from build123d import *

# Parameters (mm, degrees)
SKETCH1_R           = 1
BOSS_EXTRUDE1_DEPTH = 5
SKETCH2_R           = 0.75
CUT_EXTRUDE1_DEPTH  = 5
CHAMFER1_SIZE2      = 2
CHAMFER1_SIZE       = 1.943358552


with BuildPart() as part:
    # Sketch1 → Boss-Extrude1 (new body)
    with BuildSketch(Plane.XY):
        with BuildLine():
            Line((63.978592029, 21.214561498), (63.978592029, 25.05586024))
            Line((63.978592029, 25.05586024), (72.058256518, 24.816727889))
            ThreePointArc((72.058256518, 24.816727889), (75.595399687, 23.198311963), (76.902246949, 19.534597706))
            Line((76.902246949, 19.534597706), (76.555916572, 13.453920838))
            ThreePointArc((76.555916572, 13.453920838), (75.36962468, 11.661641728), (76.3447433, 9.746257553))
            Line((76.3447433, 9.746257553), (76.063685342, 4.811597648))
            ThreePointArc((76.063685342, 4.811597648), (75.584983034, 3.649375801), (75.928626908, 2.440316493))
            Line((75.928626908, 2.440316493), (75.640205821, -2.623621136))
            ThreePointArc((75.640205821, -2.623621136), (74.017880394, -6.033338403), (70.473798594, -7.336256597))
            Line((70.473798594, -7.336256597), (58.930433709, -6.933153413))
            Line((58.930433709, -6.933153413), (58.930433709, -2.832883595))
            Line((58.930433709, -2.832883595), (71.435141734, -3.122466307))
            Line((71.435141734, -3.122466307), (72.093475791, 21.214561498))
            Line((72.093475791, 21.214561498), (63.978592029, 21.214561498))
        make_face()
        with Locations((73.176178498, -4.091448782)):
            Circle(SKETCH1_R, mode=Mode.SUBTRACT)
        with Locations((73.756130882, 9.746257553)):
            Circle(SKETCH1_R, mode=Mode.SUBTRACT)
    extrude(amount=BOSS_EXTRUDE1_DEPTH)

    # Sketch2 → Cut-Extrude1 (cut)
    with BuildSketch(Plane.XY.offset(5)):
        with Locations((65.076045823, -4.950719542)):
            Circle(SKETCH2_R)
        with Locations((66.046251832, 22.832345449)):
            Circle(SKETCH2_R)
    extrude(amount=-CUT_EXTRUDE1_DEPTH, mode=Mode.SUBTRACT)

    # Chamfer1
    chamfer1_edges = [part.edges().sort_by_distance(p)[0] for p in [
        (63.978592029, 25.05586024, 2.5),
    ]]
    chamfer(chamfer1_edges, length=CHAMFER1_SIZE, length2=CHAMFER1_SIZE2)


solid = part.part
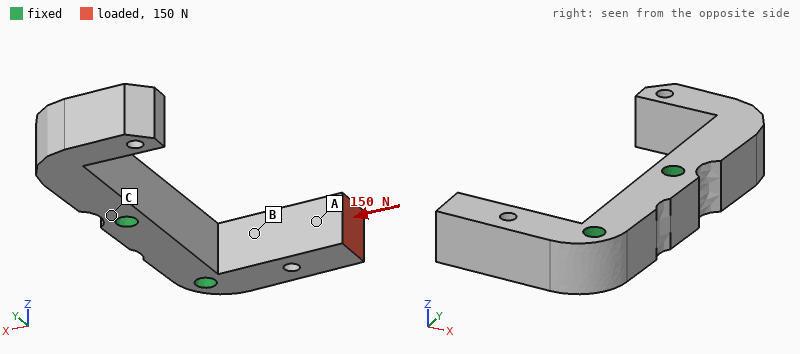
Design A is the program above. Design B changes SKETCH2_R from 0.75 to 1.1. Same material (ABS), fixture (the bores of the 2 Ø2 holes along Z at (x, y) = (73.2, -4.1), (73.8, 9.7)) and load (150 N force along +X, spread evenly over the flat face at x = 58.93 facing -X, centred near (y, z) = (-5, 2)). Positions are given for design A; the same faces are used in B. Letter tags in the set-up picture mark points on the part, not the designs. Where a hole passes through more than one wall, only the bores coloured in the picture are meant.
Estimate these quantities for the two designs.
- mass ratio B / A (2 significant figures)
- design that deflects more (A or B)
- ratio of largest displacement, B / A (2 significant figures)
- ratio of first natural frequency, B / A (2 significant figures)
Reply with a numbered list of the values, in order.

1. 0.98
2. B
3. 1.2
4. 1.0
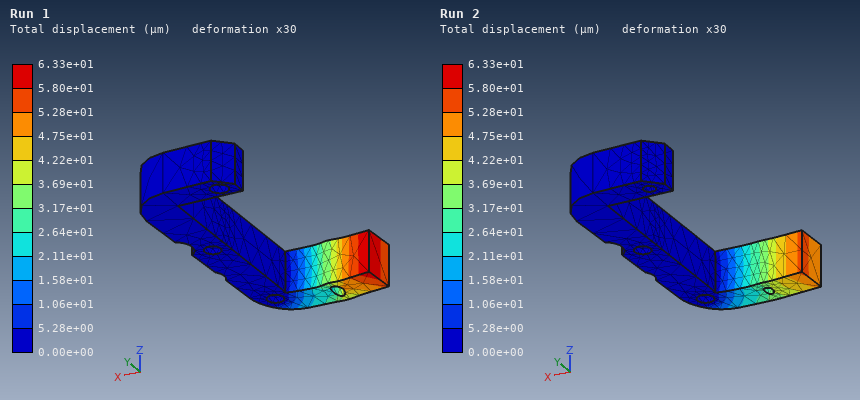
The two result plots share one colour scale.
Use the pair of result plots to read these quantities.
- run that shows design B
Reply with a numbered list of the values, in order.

1. Run 1
